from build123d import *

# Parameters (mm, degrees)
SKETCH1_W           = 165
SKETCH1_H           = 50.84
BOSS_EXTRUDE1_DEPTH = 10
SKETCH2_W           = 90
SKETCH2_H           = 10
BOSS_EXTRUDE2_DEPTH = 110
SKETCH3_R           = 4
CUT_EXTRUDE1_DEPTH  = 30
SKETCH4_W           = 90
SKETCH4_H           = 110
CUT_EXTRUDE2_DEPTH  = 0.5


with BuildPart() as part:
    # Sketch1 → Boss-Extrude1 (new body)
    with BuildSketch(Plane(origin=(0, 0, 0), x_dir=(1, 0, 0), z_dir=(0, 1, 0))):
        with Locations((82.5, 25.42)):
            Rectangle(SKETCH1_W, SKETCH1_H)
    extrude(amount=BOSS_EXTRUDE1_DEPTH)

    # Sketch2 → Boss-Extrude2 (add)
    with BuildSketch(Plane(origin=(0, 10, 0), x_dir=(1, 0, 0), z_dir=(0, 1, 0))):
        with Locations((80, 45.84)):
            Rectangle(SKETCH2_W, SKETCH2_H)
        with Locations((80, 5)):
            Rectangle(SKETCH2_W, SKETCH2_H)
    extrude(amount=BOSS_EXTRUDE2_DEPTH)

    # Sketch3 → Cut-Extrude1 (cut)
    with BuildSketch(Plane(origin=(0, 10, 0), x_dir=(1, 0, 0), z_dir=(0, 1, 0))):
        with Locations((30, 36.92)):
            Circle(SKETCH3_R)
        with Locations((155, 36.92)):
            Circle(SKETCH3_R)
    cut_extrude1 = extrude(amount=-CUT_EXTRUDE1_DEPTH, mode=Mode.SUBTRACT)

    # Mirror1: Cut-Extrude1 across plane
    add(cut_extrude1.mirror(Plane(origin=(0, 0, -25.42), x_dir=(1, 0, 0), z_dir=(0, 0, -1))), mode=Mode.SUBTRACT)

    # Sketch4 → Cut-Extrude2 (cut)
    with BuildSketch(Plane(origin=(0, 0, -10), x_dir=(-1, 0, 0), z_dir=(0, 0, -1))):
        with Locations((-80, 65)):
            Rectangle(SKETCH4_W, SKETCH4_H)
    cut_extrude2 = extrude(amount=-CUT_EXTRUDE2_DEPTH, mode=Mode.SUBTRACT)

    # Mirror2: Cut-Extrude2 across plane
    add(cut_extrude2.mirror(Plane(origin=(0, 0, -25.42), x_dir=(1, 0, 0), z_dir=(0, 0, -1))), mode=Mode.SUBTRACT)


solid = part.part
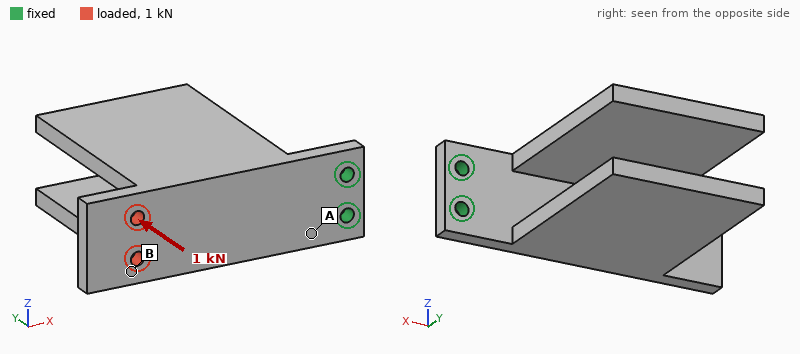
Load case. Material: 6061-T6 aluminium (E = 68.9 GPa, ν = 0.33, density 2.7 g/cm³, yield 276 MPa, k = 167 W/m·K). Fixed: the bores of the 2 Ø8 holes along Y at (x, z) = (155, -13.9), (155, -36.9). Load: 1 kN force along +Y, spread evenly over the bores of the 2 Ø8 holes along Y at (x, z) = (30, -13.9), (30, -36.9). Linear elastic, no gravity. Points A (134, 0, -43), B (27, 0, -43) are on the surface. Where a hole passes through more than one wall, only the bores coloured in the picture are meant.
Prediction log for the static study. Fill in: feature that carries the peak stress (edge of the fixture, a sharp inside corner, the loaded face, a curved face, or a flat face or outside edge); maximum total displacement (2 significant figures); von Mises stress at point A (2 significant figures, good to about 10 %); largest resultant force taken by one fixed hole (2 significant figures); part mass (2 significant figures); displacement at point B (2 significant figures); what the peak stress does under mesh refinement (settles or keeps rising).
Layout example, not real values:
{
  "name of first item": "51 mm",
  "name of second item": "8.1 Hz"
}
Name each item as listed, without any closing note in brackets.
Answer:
{
  "feature that carries the peak stress": "edge of the fixture",
  "maximum total displacement": "2.0 mm",
  "von Mises stress at point A": "120 MPa",
  "largest resultant force taken by one fixed hole": "510 N",
  "part mass": "730 g",
  "displacement at point B": "1.5 mm",
  "what the peak stress does under mesh refinement": "keeps rising"
}
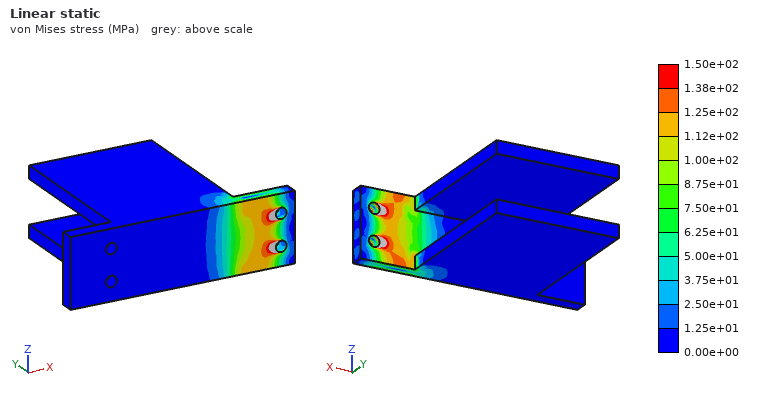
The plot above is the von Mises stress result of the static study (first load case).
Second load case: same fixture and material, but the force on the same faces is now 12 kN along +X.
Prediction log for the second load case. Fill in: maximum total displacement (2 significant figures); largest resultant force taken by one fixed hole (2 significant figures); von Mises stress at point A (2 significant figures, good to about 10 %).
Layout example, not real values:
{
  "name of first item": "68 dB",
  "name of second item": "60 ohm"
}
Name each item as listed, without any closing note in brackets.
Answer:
{
  "maximum total displacement": "88 µm",
  "largest resultant force taken by one fixed hole": "6.0 kN",
  "von Mises stress at point A": "23 MPa"
}
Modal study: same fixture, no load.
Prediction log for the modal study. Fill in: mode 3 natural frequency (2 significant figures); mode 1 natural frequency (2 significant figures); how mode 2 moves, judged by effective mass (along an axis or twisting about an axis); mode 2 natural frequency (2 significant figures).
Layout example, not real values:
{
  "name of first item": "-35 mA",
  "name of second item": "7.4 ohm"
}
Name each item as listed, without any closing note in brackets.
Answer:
{
  "mode 3 natural frequency": "510 Hz",
  "mode 1 natural frequency": "190 Hz",
  "how mode 2 moves, judged by effective mass": "along Z",
  "mode 2 natural frequency": "290 Hz"
}
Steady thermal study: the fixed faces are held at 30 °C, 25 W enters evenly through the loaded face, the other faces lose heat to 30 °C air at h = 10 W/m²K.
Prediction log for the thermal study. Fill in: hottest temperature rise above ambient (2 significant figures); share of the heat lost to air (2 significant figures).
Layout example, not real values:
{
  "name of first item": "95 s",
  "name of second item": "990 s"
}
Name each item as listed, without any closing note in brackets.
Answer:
{
  "hottest temperature rise above ambient": "22 K",
  "share of the heat lost to air": "29 %"
}
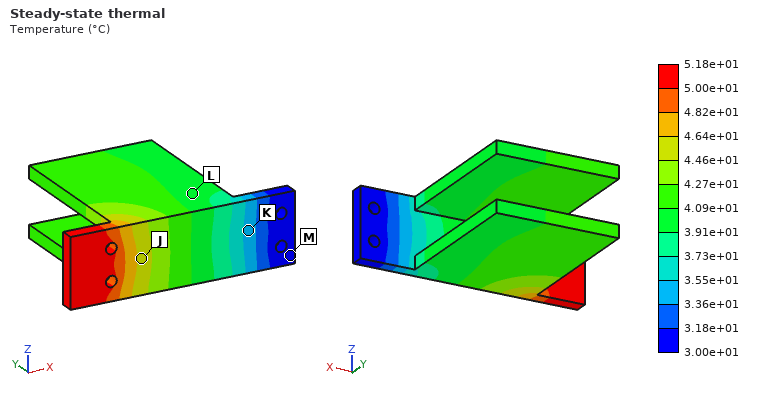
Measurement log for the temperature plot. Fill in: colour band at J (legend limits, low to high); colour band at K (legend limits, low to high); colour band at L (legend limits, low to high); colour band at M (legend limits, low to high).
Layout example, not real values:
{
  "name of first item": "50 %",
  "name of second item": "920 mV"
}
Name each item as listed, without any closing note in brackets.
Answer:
{
  "colour band at J": "4.46e+01 to 4.64e+01 °C",
  "colour band at K": "3.36e+01 to 3.55e+01 °C",
  "colour band at L": "3.91e+01 to 4.09e+01 °C",
  "colour band at M": "3.00e+01 to 3.18e+01 °C"
}
